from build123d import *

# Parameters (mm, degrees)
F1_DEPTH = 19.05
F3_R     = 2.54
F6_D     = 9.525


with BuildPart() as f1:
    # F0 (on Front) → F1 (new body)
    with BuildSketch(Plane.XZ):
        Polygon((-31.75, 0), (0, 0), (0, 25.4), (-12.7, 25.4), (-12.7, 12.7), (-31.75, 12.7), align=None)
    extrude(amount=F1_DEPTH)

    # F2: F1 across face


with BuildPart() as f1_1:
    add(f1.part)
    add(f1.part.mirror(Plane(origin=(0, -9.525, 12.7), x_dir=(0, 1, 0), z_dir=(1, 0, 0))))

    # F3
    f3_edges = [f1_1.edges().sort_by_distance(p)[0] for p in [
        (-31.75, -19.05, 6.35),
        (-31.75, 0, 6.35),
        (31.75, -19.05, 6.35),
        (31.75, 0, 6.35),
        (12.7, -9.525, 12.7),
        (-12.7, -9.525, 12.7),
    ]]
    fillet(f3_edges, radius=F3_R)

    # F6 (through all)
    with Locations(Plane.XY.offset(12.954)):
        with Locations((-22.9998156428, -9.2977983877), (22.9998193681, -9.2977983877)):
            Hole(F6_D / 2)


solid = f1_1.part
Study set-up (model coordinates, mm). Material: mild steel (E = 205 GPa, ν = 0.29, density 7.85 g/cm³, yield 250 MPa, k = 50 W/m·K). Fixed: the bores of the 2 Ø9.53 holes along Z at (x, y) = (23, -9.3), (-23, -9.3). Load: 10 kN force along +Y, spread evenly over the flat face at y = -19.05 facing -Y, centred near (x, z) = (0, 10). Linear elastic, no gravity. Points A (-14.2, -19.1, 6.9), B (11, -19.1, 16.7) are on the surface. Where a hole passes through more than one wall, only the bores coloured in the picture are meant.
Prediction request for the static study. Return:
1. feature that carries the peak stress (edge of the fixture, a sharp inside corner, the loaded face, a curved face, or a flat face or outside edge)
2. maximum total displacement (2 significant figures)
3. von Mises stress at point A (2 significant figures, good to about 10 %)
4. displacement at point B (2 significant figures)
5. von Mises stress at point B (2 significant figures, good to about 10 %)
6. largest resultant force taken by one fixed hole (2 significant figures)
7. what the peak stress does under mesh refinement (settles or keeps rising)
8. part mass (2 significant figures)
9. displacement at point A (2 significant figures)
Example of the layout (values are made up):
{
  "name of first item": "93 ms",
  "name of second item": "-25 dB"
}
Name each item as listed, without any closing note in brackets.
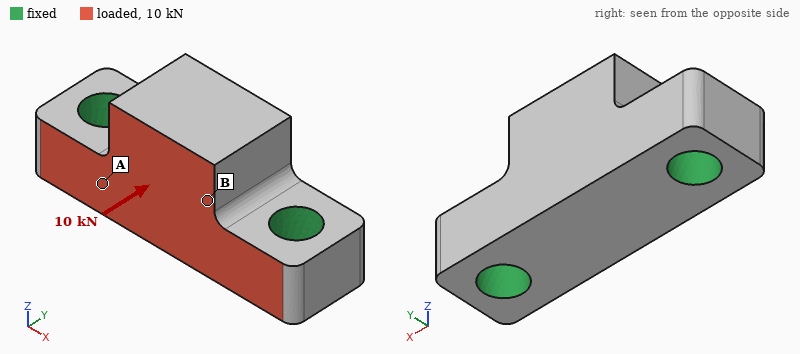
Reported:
{
  "feature that carries the peak stress": "edge of the fixture",
  "maximum total displacement": "11 µm",
  "von Mises stress at point A": "39 MPa",
  "displacement at point B": "7.5 µm",
  "von Mises stress at point B": "15 MPa",
  "largest resultant force taken by one fixed hole": "5.0 kN",
  "what the peak stress does under mesh refinement": "keeps rising",
  "part mass": "150 g",
  "displacement at point A": "3.0 µm"
}
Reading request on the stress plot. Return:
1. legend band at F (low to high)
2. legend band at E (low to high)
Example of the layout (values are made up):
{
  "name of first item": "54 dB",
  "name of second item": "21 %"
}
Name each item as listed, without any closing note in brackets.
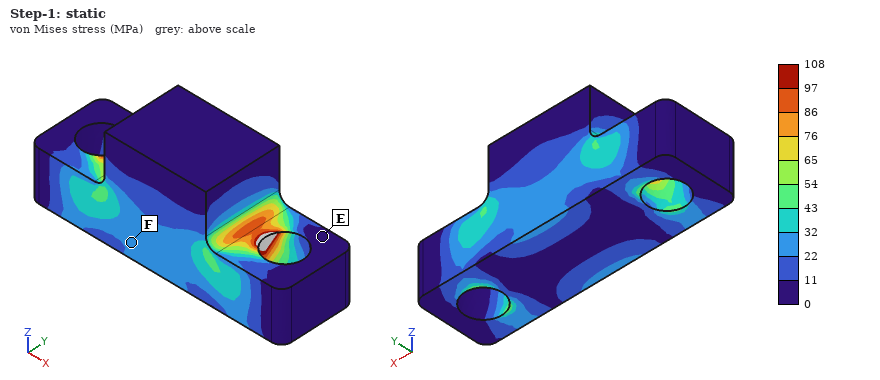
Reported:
{
  "legend band at F": "22 to 32 MPa",
  "legend band at E": "0 to 11 MPa"
}
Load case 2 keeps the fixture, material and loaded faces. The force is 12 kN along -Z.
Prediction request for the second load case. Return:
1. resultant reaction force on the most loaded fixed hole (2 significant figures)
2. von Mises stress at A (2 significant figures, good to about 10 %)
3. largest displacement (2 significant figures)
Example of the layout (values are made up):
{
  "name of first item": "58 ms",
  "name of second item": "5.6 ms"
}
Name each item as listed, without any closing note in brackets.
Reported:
{
  "resultant reaction force on the most loaded fixed hole": "6.1 kN",
  "von Mises stress at A": "100 MPa",
  "largest displacement": "18 µm"
}
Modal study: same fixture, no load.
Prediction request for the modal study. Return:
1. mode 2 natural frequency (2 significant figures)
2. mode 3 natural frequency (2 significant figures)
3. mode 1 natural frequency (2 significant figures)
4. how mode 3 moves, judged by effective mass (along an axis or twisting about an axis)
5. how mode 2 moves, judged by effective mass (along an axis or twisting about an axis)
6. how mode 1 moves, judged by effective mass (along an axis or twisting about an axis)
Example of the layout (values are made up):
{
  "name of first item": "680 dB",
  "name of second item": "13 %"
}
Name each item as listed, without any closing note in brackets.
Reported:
{
  "mode 2 natural frequency": "24 kHz",
  "mode 3 natural frequency": "29 kHz",
  "mode 1 natural frequency": "14 kHz",
  "how mode 3 moves, judged by effective mass": "along Y",
  "how mode 2 moves, judged by effective mass": "along Z",
  "how mode 1 moves, judged by effective mass": "along Y"
}
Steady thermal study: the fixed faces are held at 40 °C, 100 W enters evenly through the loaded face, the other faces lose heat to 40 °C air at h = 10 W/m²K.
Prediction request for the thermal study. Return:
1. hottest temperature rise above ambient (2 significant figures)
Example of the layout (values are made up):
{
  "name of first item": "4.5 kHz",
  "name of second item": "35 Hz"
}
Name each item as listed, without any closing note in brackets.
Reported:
{
  "hottest temperature rise above ambient": "54 K"
}
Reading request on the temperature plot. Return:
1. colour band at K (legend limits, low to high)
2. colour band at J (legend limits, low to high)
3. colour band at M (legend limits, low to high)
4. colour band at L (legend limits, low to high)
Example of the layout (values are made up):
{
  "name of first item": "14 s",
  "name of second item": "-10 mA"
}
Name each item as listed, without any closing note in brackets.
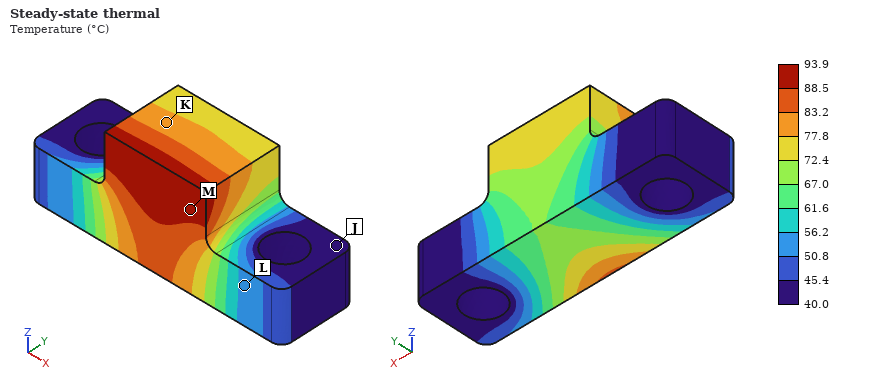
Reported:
{
  "colour band at K": "77.8 to 83.2 °C",
  "colour band at J": "40.0 to 45.4 °C",
  "colour band at M": "88.5 to 93.9 °C",
  "colour band at L": "50.8 to 56.2 °C"
}
